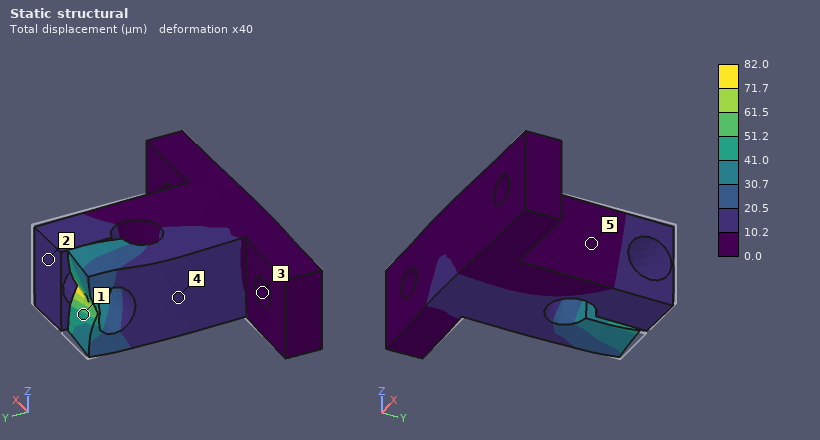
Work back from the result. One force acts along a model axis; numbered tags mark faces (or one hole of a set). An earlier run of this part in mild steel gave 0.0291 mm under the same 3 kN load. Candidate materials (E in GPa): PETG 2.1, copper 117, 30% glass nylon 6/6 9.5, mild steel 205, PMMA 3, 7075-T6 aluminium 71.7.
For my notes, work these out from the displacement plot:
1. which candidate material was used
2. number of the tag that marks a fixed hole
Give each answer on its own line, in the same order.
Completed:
7075-T6 aluminium
3
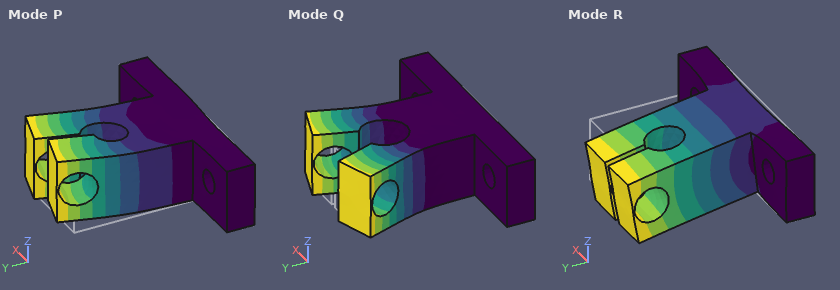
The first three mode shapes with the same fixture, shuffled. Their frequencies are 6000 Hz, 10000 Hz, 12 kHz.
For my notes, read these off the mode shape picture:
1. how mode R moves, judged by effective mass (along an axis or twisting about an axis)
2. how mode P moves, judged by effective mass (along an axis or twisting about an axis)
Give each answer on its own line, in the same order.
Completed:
along Z
along X
